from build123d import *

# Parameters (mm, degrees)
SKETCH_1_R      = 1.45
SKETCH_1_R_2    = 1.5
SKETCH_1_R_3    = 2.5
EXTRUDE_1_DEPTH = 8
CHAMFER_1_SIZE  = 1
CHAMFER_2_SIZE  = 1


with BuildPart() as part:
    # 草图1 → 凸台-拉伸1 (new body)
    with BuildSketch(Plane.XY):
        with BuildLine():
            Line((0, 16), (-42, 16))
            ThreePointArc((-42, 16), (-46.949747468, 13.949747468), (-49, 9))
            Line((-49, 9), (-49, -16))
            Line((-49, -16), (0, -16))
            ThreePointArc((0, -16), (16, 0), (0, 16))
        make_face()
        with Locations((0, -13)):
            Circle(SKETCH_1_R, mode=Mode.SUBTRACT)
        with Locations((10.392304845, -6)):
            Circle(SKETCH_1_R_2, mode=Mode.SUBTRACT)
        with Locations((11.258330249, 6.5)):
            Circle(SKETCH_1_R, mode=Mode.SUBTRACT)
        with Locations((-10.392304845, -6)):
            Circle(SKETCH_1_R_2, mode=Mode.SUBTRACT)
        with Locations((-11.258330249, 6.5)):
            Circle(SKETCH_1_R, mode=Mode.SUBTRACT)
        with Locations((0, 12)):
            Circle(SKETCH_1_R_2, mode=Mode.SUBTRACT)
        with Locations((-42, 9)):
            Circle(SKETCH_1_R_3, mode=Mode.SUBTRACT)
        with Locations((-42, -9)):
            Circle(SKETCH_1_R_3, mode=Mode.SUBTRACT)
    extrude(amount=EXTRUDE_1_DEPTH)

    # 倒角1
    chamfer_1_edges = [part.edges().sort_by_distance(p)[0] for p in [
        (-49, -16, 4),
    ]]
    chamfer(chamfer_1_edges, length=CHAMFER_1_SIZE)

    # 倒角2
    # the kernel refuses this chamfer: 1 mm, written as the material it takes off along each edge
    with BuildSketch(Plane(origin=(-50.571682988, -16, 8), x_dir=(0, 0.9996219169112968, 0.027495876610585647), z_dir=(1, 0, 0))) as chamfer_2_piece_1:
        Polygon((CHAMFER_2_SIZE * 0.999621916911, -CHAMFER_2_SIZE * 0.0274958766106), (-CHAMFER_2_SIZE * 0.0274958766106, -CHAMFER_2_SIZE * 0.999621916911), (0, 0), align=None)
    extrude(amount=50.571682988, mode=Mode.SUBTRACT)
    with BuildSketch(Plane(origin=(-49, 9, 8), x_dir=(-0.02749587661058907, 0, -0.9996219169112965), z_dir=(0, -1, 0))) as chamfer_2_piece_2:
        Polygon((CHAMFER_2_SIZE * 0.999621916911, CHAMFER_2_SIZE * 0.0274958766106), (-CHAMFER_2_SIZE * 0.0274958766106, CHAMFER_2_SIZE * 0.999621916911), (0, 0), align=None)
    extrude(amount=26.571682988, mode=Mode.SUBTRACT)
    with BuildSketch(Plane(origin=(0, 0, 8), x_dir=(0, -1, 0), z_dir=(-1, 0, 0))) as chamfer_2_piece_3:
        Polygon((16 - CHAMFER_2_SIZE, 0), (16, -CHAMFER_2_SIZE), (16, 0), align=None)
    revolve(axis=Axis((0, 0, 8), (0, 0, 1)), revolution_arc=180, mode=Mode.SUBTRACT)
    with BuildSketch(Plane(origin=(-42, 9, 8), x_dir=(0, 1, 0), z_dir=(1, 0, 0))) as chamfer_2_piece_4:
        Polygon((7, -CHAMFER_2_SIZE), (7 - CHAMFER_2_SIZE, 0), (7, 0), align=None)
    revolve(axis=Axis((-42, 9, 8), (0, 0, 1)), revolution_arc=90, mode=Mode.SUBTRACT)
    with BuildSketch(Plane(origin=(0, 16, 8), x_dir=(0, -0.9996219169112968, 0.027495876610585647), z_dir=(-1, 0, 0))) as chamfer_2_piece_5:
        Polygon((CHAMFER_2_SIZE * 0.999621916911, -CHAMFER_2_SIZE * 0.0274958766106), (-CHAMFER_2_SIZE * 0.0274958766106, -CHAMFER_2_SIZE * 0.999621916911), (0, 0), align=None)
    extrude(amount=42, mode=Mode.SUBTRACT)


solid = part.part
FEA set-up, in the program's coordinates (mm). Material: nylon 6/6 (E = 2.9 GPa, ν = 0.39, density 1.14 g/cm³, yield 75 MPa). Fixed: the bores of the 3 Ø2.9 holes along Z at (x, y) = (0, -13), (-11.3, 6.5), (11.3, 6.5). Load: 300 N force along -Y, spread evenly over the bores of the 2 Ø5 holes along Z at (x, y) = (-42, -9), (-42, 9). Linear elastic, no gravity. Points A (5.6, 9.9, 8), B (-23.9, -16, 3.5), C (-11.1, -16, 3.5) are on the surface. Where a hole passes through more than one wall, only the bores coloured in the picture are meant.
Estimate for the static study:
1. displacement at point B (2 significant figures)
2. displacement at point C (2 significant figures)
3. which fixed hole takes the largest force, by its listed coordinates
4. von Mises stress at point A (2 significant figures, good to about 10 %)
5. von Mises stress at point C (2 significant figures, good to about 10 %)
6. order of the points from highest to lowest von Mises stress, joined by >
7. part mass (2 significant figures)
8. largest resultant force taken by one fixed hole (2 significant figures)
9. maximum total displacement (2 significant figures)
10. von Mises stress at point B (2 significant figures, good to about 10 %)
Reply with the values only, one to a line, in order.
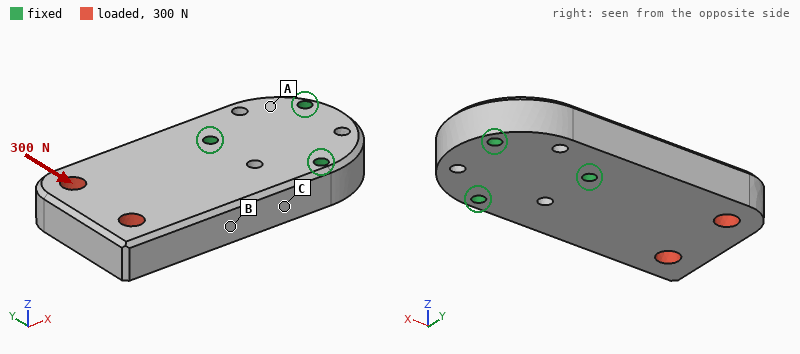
0.077 mm
0.032 mm
(-11.3, 6.5)
1.3 MPa
6.9 MPa
C > B > A
17 g
480 N
0.18 mm
4.6 MPa
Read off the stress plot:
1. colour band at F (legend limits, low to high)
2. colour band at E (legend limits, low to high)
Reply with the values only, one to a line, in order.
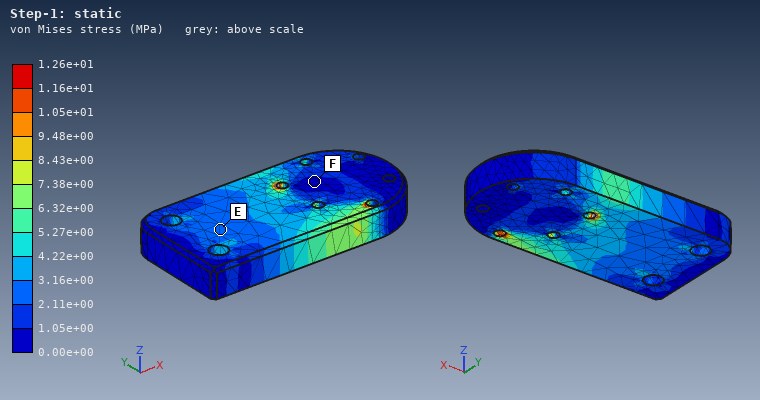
0.00e+00 to 1.05e+00 MPa
2.11e+00 to 3.16e+00 MPa
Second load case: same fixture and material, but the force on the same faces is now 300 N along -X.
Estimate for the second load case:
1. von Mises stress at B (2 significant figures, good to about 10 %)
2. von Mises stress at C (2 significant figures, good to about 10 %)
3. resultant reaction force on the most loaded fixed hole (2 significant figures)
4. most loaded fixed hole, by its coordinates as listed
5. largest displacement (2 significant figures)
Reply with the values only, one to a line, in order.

1.2 MPa
1.4 MPa
160 N
(-11.3, 6.5)
22 µm
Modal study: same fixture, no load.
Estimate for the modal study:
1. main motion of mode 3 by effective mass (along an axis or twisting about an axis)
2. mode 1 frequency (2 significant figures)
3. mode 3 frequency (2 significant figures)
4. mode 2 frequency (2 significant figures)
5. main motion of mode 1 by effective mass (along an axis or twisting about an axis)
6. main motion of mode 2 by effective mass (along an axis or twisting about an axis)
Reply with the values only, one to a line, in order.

along Y
1200 Hz
3200 Hz
3000 Hz
along Z
twisting about X
